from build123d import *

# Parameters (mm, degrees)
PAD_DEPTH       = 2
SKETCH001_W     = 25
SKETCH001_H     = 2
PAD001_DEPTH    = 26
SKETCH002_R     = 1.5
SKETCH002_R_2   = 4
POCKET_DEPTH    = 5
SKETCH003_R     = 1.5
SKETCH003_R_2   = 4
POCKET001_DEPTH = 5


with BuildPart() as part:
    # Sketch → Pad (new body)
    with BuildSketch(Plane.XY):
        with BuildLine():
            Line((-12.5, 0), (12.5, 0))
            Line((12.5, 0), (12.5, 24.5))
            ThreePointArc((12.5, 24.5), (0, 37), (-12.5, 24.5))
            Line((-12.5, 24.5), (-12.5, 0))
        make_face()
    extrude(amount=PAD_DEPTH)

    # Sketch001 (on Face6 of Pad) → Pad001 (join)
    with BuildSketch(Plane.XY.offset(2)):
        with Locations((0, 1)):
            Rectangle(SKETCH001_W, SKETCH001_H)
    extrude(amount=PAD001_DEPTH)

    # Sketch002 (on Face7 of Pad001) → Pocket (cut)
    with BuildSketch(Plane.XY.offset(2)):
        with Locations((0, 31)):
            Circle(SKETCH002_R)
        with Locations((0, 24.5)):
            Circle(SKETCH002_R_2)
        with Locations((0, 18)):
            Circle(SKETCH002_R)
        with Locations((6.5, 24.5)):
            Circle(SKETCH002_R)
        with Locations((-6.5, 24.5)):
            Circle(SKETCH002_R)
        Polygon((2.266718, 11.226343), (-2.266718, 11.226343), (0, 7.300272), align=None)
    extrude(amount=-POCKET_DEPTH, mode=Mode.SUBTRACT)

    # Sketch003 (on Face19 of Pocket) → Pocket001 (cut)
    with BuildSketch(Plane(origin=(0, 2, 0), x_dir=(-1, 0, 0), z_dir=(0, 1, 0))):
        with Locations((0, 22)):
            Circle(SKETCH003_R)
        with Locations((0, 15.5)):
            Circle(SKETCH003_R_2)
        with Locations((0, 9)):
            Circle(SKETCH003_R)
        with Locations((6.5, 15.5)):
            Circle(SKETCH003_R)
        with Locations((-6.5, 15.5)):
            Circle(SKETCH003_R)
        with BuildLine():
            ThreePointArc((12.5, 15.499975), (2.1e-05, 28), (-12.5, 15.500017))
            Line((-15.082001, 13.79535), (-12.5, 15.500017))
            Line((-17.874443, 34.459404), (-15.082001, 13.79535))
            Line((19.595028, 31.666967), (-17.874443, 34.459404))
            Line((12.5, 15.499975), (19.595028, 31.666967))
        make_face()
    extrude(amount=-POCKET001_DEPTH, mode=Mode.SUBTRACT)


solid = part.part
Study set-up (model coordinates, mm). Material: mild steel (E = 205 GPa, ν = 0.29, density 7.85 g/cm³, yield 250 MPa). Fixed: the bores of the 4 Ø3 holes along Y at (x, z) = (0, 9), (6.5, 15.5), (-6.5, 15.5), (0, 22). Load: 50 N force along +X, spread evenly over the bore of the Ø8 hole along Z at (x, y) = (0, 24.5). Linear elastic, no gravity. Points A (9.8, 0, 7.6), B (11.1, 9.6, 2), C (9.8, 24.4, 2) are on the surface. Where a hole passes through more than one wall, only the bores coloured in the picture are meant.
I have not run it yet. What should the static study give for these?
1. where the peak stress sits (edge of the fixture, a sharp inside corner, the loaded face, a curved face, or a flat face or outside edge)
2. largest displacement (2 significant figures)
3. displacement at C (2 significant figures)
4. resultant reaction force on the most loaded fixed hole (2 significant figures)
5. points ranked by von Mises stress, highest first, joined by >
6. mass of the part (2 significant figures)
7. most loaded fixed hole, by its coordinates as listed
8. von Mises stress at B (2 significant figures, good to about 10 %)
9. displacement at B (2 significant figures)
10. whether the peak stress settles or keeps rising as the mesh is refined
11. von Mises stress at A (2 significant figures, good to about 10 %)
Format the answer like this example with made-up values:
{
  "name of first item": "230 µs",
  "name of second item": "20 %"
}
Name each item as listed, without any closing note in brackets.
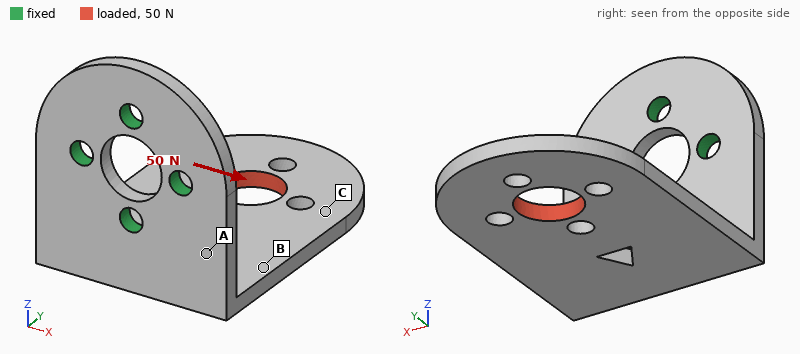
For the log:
{
  "where the peak stress sits": "edge of the fixture",
  "largest displacement": "47 µm",
  "displacement at C": "34 µm",
  "resultant reaction force on the most loaded fixed hole": "49 N",
  "points ranked by von Mises stress, highest first, joined by >": "A > B > C",
  "mass of the part": "20 g",
  "most loaded fixed hole, by its coordinates as listed": "(0, 9)",
  "von Mises stress at B": "13 MPa",
  "displacement at B": "19 µm",
  "whether the peak stress settles or keeps rising as the mesh is refined": "keeps rising",
  "von Mises stress at A": "26 MPa"
}
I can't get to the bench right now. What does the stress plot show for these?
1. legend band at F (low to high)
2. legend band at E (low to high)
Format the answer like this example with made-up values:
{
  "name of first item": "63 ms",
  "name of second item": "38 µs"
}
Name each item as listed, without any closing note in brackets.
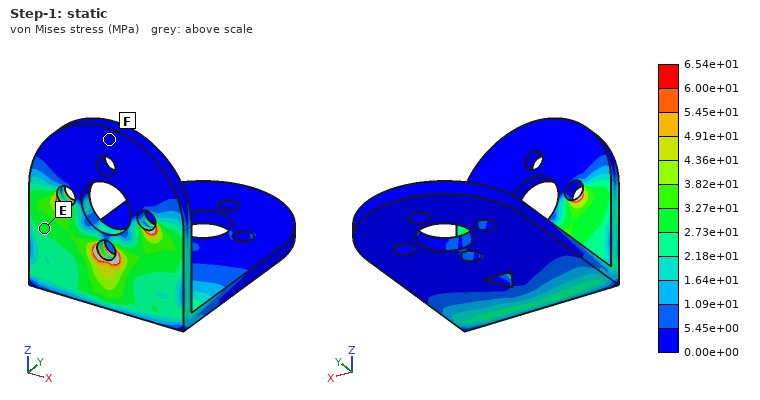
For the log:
{
  "legend band at F": "0.00e+00 to 5.45e+00 MPa",
  "legend band at E": "2.73e+01 to 3.27e+01 MPa"
}
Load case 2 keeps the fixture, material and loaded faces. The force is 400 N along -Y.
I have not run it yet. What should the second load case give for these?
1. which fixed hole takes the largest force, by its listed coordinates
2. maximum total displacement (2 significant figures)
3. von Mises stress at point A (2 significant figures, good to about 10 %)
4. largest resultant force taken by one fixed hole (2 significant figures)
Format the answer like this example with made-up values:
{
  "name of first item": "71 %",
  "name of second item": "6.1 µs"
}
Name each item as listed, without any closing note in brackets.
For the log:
{
  "which fixed hole takes the largest force, by its listed coordinates": "(0, 9)",
  "maximum total displacement": "0.15 mm",
  "von Mises stress at point A": "69 MPa",
  "largest resultant force taken by one fixed hole": "510 N"
}
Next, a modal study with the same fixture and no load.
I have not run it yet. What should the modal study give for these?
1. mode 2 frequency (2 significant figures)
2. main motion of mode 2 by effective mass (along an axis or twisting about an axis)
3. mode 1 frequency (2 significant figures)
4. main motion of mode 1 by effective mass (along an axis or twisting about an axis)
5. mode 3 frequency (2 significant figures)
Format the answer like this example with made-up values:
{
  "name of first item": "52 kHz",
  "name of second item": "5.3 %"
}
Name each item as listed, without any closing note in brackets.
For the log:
{
  "mode 2 frequency": "2100 Hz",
  "main motion of mode 2 by effective mass": "along X",
  "mode 1 frequency": "1100 Hz",
  "main motion of mode 1 by effective mass": "along Z",
  "mode 3 frequency": "4500 Hz"
}
